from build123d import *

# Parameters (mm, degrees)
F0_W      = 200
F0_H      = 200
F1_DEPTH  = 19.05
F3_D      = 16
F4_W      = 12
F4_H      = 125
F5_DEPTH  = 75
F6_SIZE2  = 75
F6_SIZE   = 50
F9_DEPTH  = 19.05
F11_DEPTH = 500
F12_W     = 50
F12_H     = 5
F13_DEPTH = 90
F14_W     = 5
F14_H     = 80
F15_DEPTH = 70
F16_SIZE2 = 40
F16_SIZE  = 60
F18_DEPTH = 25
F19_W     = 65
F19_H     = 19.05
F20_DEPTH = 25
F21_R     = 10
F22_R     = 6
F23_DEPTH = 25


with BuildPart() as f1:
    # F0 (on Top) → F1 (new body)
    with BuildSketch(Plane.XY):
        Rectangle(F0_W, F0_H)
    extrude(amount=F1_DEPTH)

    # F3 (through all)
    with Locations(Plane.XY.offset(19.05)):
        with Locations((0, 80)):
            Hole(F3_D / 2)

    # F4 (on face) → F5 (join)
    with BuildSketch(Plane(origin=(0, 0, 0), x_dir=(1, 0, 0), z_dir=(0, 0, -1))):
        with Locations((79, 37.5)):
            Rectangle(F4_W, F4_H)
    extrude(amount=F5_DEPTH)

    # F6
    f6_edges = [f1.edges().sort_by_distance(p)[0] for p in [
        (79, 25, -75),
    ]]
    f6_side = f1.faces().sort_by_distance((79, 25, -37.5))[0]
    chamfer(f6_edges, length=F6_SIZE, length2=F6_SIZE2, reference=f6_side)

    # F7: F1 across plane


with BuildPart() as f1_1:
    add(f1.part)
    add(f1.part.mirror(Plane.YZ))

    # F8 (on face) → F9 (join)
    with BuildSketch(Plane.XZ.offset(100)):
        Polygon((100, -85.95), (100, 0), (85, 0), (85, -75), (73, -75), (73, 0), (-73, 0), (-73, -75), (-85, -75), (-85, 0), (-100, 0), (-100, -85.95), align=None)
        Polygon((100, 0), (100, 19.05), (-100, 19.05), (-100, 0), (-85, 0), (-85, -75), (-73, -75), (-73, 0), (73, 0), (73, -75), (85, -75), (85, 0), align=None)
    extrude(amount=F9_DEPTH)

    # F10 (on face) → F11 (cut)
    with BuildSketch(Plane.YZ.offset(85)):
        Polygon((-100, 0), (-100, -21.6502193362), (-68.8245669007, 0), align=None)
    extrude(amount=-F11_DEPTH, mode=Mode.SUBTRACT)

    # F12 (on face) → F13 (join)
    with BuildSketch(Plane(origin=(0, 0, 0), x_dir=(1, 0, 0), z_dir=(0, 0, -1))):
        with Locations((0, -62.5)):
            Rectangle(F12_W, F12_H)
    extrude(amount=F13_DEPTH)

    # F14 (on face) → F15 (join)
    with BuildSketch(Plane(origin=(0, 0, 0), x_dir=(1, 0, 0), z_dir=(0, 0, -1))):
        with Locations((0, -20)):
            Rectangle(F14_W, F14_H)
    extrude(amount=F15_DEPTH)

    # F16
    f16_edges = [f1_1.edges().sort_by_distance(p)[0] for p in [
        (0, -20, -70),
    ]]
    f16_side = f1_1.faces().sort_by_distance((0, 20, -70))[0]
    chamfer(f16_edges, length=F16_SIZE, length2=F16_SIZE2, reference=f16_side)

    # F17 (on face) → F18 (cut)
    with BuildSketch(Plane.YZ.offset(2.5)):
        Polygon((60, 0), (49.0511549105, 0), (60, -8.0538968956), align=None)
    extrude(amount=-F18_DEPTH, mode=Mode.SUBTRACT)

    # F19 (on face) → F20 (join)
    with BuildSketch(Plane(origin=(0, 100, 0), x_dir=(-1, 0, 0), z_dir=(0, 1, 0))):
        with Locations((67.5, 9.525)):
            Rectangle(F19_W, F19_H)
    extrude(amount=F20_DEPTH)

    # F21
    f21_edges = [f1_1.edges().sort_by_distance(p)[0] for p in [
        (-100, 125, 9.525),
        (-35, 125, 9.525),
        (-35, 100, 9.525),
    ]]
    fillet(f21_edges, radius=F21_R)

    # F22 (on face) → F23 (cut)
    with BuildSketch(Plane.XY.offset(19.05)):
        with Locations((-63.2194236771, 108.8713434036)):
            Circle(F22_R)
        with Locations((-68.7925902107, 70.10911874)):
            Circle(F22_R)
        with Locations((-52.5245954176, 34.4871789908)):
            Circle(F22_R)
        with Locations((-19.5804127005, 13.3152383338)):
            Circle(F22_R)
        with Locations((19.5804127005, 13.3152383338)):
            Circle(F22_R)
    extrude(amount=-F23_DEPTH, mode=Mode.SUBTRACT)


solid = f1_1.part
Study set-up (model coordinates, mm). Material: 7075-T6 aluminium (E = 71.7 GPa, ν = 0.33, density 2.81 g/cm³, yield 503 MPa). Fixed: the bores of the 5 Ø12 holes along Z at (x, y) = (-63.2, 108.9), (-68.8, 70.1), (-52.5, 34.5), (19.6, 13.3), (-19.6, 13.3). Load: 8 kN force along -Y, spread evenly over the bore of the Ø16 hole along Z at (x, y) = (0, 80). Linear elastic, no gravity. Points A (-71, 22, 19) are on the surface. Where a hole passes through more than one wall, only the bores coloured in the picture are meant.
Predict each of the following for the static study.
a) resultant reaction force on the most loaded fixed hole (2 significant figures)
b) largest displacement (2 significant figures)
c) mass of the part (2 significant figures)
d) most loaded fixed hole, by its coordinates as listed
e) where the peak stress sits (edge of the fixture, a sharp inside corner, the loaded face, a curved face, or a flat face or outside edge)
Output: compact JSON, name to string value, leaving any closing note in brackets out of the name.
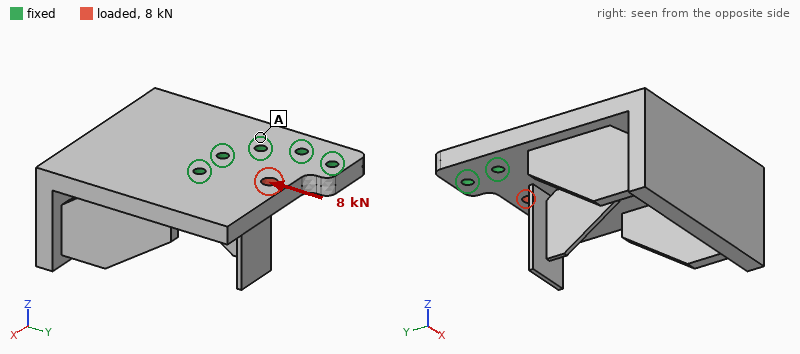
{"resultant reaction force on the most loaded fixed hole": "3.9 kN", "largest displacement": "8.3 µm", "mass of the part": "3.9 kg", "most loaded fixed hole, by its coordinates as listed": "(19.6, 13.3)", "where the peak stress sits": "the loaded face"}
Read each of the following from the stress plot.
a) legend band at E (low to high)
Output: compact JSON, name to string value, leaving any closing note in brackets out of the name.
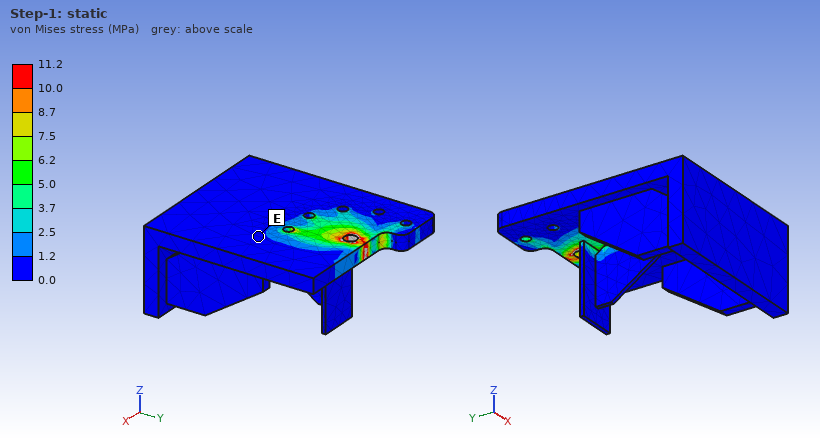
{"legend band at E": "0.0 to 1.2 MPa"}
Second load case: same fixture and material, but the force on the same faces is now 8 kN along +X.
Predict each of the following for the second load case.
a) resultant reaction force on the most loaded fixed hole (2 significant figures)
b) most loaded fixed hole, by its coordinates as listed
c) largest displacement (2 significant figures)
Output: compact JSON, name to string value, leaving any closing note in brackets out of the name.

{"resultant reaction force on the most loaded fixed hole": "2.8 kN", "most loaded fixed hole, by its coordinates as listed": "(-68.8, 70.1)", "largest displacement": "8.1 µm"}
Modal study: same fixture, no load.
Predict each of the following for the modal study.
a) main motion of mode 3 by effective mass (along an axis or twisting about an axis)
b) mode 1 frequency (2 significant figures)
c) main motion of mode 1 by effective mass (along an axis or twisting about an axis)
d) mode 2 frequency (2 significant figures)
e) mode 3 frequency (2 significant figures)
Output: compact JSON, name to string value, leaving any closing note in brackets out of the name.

{"main motion of mode 3 by effective mass": "along Z", "mode 1 frequency": "500 Hz", "main motion of mode 1 by effective mass": "along Z", "mode 2 frequency": "660 Hz", "mode 3 frequency": "1600 Hz"}
